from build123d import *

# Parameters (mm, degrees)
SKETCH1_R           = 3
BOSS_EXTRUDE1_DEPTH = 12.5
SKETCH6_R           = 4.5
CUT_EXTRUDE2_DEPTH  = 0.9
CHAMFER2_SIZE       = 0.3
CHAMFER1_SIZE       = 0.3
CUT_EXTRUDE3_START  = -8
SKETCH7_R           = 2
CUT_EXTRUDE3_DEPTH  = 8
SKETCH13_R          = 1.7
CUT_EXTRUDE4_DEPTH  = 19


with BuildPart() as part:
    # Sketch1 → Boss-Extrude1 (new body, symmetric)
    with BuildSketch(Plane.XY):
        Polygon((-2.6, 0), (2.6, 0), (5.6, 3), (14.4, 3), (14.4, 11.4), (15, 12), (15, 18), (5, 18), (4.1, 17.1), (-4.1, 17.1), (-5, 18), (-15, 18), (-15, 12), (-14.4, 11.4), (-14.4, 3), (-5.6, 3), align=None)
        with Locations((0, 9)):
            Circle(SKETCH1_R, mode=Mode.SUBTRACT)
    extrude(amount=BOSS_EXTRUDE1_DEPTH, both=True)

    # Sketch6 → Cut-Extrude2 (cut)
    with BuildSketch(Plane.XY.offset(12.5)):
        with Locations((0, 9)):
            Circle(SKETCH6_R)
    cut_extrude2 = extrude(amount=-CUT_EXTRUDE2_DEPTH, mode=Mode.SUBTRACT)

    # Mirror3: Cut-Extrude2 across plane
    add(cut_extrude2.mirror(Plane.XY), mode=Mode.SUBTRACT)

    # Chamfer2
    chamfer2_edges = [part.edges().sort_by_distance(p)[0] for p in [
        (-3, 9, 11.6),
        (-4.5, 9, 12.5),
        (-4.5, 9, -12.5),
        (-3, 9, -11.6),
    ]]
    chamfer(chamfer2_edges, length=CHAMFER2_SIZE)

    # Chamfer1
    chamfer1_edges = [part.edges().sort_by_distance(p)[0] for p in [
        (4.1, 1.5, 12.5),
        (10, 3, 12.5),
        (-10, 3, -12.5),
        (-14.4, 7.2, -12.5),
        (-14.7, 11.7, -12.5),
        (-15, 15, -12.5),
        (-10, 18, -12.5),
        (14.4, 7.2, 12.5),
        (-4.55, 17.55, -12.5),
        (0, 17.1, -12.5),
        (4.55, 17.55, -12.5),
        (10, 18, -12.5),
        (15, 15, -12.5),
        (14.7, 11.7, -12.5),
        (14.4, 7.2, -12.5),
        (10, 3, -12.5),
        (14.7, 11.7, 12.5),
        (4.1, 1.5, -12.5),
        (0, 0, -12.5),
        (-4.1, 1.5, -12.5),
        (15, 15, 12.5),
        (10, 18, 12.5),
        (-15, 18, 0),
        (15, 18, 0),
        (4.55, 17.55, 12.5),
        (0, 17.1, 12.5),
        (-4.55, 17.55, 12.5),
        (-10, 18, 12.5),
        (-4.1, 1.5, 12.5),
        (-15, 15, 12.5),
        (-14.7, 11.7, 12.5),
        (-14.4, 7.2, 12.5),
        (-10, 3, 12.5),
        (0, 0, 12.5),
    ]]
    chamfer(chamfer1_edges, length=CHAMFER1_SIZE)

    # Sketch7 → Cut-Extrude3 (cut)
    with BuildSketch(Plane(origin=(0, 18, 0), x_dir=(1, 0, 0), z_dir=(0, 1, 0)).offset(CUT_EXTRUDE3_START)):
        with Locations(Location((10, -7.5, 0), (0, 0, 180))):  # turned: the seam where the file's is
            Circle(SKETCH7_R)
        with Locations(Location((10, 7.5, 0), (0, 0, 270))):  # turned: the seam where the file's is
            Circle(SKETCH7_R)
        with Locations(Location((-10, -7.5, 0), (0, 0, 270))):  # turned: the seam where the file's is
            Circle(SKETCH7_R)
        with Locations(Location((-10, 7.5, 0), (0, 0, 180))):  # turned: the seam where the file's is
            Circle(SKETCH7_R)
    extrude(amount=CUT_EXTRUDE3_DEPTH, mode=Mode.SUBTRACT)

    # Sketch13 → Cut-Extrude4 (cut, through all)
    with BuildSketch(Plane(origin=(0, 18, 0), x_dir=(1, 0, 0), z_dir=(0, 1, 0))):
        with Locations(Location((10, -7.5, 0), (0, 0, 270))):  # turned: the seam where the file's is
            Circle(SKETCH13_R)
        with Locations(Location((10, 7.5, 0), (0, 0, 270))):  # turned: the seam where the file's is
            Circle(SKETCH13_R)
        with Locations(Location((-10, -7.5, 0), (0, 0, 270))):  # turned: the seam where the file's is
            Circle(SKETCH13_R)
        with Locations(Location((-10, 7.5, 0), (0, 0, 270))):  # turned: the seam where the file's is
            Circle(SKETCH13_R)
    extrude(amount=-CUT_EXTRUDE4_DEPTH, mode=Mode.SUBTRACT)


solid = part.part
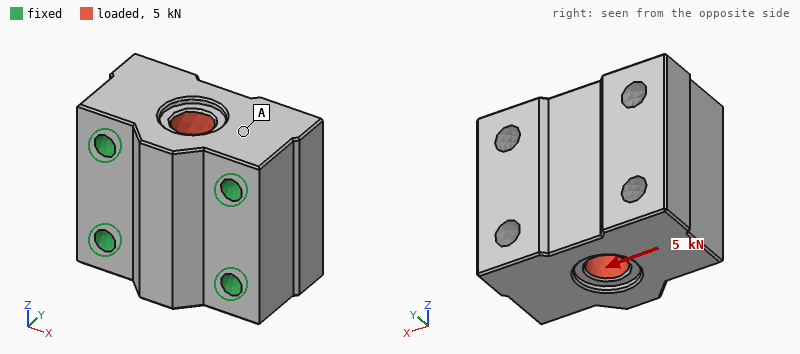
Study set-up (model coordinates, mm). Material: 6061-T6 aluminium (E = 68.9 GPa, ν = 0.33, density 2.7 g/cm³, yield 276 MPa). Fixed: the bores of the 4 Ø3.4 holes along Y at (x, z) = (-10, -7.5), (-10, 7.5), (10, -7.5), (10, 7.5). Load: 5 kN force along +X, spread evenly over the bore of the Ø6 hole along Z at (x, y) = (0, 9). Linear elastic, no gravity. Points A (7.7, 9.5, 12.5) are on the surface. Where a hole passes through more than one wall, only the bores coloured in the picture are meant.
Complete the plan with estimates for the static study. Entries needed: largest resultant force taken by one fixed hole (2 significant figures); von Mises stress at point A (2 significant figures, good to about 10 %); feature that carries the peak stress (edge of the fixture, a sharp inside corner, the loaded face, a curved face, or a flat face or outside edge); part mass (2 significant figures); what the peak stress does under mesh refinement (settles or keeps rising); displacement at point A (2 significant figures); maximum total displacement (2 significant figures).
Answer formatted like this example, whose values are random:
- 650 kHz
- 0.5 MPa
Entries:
- 1.3 kN
- 6.3 MPa
- edge of the fixture
- 27 g
- keeps rising
- 1.1 µm
- 2.8 µm
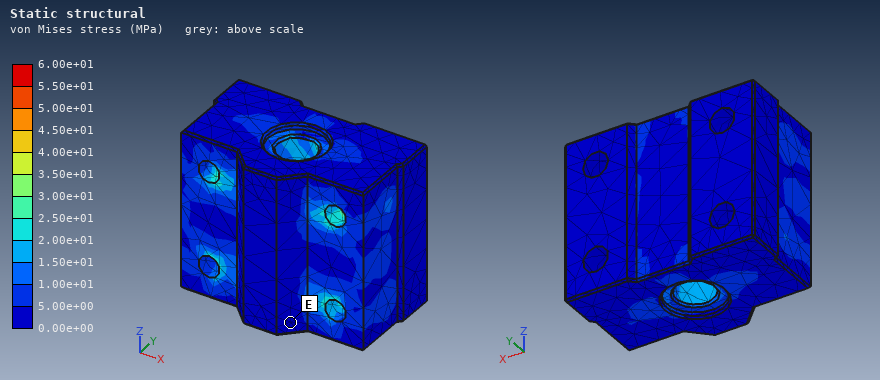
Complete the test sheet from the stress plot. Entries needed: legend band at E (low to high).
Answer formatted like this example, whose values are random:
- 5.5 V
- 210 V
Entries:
- 0.00e+00 to 5.00e+00 MPa
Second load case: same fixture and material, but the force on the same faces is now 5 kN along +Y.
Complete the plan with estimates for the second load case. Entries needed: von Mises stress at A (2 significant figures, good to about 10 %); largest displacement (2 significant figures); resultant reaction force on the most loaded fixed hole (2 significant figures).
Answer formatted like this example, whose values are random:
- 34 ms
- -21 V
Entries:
- 12 MPa
- 4.3 µm
- 1.3 kN
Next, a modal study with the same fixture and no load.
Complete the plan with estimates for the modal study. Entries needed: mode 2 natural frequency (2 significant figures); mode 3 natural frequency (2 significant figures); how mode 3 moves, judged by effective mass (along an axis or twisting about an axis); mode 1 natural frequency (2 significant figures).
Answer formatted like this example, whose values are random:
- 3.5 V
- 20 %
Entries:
- 46 kHz
- 54 kHz
- along Y
- 45 kHz
